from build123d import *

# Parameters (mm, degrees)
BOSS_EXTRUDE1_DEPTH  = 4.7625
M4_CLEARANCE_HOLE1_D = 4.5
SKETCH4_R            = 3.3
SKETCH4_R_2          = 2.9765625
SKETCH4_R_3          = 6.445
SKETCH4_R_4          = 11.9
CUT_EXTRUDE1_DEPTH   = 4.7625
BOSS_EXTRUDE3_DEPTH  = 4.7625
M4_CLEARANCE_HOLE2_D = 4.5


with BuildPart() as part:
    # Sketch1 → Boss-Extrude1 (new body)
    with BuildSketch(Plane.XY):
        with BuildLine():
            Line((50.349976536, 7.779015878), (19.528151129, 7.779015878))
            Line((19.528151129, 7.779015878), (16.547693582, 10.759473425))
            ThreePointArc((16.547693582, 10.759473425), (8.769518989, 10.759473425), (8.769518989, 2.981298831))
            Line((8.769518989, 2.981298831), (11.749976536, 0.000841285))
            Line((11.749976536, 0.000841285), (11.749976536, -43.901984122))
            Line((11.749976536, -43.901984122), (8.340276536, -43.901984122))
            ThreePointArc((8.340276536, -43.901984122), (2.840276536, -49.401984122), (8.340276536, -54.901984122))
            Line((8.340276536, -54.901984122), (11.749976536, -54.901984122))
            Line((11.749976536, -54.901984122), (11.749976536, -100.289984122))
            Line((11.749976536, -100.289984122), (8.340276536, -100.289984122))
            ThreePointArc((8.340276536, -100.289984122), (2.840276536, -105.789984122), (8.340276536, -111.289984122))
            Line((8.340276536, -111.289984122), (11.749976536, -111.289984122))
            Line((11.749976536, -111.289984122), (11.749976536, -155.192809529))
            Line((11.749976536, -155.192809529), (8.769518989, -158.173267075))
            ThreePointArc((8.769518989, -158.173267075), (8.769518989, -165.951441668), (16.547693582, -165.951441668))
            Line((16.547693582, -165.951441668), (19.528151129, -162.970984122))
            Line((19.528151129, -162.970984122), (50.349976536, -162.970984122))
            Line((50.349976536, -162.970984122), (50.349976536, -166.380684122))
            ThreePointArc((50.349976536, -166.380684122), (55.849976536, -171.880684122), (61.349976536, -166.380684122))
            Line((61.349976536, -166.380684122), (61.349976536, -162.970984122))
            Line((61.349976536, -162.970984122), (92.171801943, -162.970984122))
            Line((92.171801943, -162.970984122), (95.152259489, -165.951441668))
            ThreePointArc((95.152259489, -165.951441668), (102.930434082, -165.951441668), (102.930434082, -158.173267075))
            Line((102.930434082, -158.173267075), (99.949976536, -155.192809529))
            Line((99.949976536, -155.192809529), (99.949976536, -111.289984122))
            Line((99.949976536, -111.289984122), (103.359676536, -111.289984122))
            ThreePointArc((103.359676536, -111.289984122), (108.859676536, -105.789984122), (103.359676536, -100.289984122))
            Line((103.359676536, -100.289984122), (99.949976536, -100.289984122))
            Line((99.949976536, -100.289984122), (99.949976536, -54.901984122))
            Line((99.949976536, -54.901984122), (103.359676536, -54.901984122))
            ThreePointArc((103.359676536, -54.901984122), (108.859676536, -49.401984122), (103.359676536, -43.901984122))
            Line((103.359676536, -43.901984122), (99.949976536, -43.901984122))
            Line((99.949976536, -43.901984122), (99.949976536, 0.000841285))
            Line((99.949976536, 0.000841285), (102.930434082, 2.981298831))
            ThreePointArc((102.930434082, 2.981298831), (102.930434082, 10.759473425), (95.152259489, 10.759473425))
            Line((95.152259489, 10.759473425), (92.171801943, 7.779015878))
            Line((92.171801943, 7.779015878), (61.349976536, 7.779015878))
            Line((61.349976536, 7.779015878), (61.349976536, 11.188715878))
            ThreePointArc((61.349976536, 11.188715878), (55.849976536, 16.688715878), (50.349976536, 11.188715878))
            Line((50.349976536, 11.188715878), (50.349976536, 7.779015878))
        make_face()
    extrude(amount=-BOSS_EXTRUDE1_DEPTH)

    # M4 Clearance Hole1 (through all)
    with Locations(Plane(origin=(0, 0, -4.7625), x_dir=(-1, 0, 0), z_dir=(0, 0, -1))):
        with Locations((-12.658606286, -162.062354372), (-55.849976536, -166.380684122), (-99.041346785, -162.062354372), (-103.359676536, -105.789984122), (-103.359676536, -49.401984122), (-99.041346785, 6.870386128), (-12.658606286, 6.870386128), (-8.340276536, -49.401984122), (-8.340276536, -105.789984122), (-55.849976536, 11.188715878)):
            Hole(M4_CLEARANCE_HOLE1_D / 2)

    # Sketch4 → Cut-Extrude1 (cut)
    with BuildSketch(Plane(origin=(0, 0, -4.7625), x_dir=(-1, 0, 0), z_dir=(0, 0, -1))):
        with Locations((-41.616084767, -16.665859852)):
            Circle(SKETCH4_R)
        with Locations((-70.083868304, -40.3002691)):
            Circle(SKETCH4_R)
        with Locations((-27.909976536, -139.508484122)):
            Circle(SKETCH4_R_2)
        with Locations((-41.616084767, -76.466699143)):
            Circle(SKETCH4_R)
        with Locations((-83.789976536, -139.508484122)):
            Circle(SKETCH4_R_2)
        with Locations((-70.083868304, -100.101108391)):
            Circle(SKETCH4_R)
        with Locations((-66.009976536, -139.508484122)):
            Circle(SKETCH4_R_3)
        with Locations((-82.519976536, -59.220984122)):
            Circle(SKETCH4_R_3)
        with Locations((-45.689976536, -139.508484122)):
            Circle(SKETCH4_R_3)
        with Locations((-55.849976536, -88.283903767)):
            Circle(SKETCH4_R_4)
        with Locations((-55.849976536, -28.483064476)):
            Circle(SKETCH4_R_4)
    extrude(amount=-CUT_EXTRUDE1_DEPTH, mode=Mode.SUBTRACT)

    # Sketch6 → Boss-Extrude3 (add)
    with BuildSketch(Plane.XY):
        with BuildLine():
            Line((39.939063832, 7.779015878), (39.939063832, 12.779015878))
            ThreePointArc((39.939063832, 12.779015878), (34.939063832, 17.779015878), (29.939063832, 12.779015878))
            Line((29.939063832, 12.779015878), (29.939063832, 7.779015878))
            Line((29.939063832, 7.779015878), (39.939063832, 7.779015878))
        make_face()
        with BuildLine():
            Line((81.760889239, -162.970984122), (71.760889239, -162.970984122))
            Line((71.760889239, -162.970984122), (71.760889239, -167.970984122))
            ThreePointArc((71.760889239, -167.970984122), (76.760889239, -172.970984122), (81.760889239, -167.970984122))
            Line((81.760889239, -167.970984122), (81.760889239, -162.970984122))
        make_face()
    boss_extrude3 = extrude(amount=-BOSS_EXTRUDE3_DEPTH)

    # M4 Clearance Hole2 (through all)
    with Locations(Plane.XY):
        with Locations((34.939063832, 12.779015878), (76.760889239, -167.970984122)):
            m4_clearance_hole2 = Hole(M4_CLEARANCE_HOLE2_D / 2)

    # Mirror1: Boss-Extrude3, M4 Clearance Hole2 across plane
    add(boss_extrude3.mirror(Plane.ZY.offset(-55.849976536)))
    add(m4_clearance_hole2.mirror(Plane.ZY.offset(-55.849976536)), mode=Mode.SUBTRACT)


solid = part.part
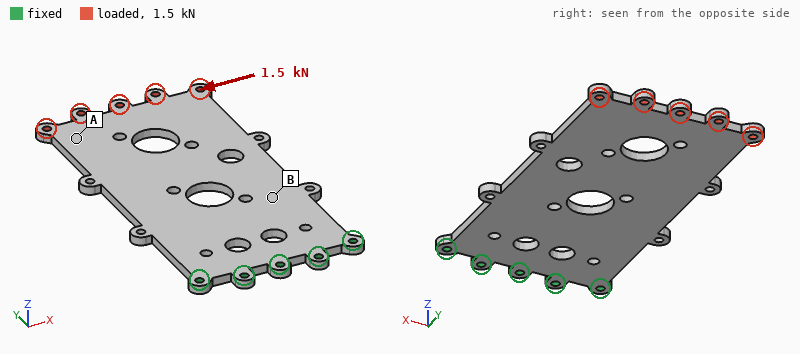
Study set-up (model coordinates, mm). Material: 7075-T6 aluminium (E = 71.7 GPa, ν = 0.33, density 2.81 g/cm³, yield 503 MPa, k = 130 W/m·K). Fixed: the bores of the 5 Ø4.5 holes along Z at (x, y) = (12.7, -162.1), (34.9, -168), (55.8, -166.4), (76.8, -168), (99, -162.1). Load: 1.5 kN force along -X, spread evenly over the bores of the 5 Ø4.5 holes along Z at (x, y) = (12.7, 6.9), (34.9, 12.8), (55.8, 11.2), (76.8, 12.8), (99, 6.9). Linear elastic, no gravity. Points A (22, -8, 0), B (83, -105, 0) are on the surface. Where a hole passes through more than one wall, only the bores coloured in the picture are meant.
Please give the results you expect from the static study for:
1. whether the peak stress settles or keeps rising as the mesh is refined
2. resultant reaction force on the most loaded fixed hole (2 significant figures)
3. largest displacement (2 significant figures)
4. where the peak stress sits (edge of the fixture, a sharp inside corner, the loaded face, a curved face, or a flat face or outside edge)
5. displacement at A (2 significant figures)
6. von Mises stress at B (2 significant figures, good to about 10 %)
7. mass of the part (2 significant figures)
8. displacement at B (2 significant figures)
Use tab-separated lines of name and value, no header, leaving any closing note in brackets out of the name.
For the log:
whether the peak stress settles or keeps rising as the mesh is refined	keeps rising
resultant reaction force on the most loaded fixed hole	2.6 kN
largest displacement	0.21 mm
where the peak stress sits	edge of the fixture
displacement at A	0.17 mm
von Mises stress at B	21 MPa
mass of the part	190 g
displacement at B	0.039 mm
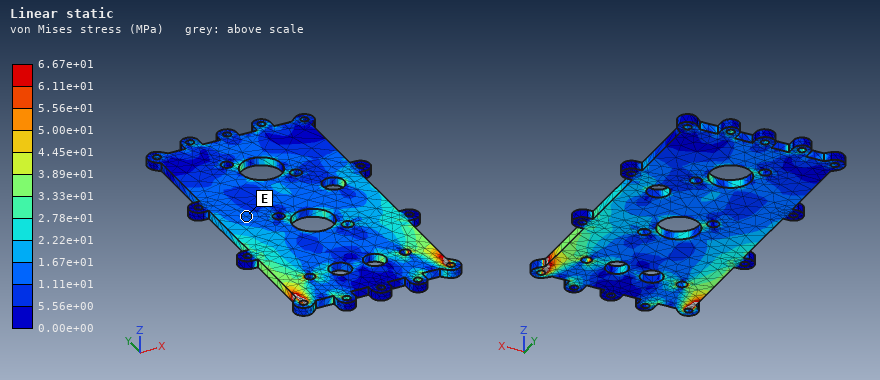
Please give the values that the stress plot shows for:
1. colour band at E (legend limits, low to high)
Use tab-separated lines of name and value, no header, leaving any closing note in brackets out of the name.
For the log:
colour band at E	1.11e+01 to 1.67e+01 MPa
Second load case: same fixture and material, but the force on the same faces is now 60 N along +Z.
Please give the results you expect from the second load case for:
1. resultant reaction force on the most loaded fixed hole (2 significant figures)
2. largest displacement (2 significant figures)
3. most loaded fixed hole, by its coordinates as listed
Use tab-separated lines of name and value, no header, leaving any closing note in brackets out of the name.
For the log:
resultant reaction force on the most loaded fixed hole	72 N
largest displacement	2.5 mm
most loaded fixed hole, by its coordinates as listed	(55.8, -166.4)
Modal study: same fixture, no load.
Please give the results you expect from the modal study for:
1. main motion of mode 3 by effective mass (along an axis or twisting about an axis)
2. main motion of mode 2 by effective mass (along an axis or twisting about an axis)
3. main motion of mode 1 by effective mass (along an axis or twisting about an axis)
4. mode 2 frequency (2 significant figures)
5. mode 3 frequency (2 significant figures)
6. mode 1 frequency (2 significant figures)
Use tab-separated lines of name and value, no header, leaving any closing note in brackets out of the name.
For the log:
main motion of mode 3 by effective mass	along Z
main motion of mode 2 by effective mass	twisting about Y
main motion of mode 1 by effective mass	along Z
mode 2 frequency	490 Hz
mode 3 frequency	720 Hz
mode 1 frequency	120 Hz
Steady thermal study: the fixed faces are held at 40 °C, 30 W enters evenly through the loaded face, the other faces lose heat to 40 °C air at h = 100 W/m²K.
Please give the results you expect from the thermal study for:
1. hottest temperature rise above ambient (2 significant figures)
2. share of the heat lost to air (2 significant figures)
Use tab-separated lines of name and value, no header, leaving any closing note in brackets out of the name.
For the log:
hottest temperature rise above ambient	35 K
share of the heat lost to air	95 %
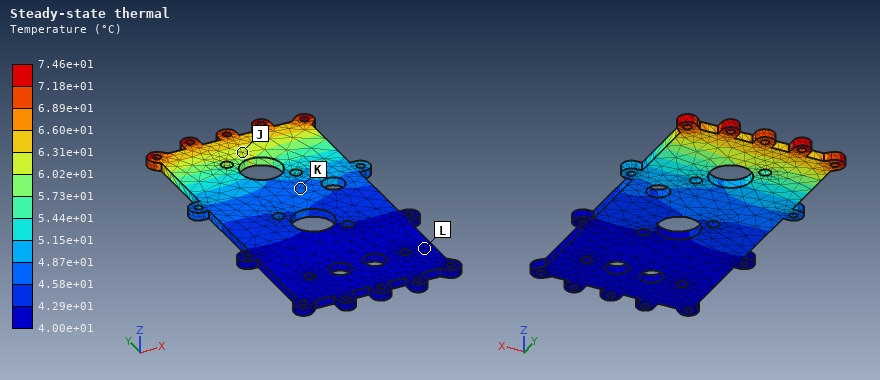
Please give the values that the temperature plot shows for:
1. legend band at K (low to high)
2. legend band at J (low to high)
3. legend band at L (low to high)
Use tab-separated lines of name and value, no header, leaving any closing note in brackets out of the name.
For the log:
legend band at K	4.58e+01 to 4.87e+01 °C
legend band at J	6.02e+01 to 6.31e+01 °C
legend band at L	4.00e+01 to 4.29e+01 °C
